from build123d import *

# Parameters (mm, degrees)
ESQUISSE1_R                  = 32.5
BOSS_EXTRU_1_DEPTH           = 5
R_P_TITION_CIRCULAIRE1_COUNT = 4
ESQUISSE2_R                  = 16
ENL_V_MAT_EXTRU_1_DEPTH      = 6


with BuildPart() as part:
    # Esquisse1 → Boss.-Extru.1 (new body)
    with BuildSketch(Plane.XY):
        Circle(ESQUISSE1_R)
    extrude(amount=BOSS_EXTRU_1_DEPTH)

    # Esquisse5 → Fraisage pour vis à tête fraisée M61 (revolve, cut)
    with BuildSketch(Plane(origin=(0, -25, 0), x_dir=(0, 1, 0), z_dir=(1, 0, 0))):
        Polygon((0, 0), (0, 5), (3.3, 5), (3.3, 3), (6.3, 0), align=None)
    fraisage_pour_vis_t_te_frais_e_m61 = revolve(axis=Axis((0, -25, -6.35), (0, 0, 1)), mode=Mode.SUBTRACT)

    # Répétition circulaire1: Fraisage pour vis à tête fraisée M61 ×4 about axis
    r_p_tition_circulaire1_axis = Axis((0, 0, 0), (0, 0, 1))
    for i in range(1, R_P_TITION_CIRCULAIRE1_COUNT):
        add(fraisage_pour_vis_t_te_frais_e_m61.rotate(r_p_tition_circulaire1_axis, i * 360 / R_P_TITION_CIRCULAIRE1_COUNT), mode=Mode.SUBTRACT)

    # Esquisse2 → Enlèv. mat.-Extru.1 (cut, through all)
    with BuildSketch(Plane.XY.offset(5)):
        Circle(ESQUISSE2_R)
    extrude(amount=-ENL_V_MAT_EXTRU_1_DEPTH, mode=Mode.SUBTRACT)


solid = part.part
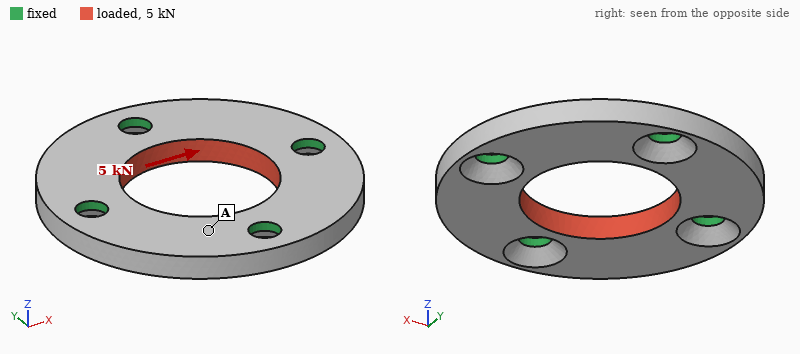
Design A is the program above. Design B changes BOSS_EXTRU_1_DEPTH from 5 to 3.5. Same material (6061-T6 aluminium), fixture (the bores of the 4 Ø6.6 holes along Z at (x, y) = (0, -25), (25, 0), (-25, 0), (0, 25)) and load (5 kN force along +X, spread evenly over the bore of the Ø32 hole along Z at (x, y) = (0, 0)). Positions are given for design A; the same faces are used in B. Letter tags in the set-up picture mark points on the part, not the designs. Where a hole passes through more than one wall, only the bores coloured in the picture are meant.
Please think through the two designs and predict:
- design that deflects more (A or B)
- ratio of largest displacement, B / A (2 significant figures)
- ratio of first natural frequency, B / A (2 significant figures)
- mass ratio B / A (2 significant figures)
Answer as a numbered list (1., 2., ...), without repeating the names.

1. B
2. 3.7
3. 0.63
4. 0.69
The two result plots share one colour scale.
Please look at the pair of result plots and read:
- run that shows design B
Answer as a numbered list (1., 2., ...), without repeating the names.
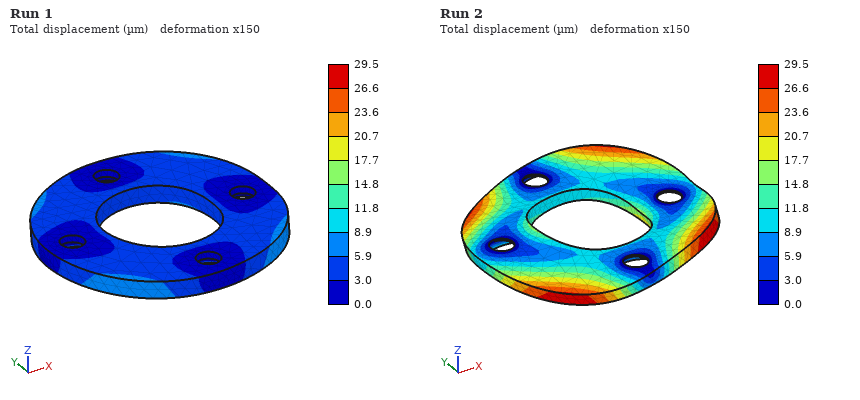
1. Run 2
